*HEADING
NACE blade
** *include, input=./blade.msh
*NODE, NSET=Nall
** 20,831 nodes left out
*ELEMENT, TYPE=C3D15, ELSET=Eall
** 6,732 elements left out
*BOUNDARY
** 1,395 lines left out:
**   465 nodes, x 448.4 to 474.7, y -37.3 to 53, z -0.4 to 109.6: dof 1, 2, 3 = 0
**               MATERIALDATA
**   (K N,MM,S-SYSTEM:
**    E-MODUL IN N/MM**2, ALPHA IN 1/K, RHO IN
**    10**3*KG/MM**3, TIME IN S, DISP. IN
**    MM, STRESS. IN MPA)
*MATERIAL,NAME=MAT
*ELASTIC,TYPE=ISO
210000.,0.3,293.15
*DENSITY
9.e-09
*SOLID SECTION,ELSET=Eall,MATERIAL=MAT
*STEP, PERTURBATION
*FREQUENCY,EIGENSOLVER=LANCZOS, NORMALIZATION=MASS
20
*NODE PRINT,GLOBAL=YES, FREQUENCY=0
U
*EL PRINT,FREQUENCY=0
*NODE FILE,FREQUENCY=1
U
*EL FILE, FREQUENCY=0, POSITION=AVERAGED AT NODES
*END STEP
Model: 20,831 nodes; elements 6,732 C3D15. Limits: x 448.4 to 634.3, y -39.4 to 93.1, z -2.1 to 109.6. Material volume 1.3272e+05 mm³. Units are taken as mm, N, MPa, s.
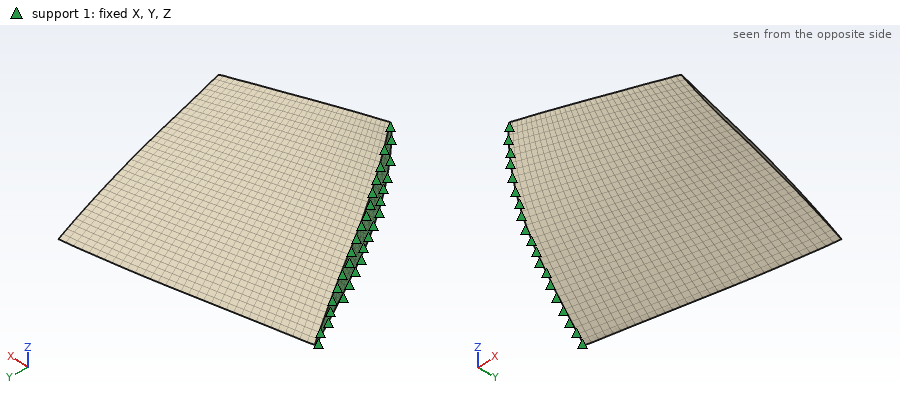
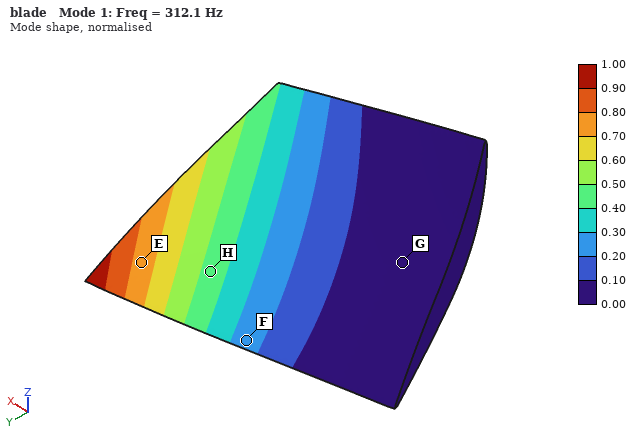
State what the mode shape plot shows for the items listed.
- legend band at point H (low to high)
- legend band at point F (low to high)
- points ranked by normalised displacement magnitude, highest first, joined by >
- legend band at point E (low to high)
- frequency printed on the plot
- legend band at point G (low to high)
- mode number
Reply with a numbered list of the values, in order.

1. 0.40 to 0.50
2. 0.20 to 0.30
3. E > H > F > G
4. 0.70 to 0.80
5. 312.1 Hz
6. 0.00 to 0.10
7. 1
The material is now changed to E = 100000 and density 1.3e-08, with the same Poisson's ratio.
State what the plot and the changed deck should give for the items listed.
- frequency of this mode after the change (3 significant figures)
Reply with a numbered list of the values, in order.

1. 179 Hz
